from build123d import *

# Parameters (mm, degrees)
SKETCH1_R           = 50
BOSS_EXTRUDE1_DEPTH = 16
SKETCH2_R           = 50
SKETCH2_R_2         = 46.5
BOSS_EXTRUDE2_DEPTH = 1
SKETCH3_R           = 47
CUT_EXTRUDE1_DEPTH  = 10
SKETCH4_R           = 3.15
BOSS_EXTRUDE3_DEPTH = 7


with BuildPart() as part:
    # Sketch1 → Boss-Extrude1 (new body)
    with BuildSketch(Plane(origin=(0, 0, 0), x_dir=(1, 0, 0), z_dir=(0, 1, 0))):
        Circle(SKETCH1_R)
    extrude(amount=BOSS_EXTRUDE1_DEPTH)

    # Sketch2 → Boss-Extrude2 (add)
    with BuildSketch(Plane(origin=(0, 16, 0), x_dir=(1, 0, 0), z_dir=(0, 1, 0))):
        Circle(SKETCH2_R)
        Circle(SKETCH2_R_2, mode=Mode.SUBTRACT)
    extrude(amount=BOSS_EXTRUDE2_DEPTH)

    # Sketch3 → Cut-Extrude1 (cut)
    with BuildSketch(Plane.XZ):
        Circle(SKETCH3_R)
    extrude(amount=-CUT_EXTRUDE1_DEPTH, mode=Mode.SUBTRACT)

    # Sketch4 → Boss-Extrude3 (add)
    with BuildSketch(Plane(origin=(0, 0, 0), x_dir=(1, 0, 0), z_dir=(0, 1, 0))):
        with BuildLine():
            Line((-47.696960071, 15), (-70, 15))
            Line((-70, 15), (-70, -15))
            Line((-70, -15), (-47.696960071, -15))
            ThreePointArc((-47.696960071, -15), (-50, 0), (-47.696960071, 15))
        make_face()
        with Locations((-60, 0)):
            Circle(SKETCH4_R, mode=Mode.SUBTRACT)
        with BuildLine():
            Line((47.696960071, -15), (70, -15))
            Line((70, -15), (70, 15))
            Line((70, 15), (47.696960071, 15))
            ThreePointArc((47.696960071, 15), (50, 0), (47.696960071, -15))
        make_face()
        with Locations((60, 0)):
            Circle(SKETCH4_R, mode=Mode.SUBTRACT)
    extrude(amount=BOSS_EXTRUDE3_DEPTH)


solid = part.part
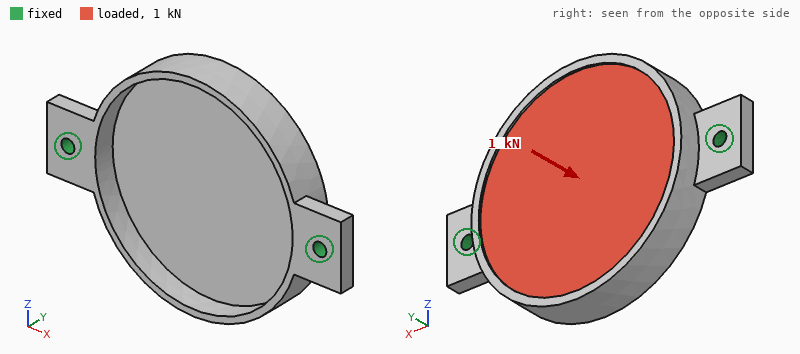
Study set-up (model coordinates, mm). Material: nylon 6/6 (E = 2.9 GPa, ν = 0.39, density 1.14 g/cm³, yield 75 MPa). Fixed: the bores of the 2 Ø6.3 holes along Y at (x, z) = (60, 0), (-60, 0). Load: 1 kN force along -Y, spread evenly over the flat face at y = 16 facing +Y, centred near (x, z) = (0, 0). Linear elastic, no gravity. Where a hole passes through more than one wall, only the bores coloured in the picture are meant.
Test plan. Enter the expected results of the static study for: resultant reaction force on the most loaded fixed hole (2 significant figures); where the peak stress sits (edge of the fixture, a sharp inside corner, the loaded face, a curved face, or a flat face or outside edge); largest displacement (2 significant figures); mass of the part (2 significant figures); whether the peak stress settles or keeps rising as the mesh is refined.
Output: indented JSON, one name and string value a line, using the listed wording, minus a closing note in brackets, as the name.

{
  "resultant reaction force on the most loaded fixed hole": "990 N",
  "where the peak stress sits": "edge of the fixture",
  "largest displacement": "0.95 mm",
  "mass of the part": "75 g",
  "whether the peak stress settles or keeps rising as the mesh is refined": "keeps rising"
}
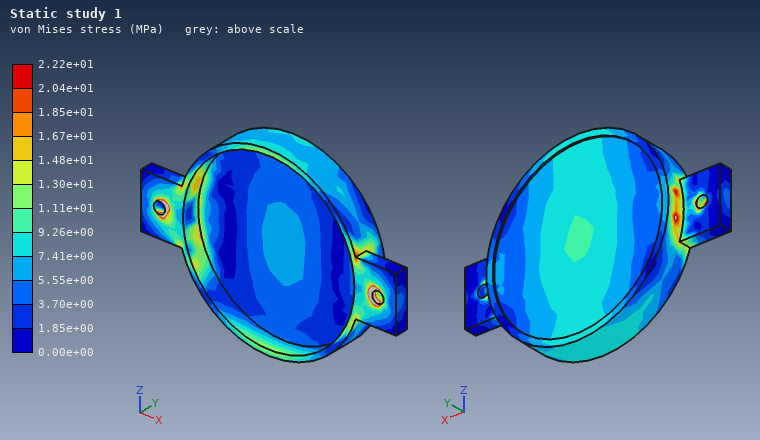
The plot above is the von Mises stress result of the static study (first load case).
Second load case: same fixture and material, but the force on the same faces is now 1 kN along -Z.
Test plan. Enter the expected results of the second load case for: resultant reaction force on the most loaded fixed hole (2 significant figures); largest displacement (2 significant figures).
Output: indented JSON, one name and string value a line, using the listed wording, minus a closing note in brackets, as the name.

{
  "resultant reaction force on the most loaded fixed hole": "500 N",
  "largest displacement": "1.6 mm"
}
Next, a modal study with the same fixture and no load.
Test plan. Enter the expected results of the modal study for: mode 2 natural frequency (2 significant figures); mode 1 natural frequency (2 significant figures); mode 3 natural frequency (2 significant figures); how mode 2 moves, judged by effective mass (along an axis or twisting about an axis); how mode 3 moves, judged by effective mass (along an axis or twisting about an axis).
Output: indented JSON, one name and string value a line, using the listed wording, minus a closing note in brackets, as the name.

{
  "mode 2 natural frequency": "760 Hz",
  "mode 1 natural frequency": "440 Hz",
  "mode 3 natural frequency": "1300 Hz",
  "how mode 2 moves, judged by effective mass": "along Y",
  "how mode 3 moves, judged by effective mass": "along X"
}
